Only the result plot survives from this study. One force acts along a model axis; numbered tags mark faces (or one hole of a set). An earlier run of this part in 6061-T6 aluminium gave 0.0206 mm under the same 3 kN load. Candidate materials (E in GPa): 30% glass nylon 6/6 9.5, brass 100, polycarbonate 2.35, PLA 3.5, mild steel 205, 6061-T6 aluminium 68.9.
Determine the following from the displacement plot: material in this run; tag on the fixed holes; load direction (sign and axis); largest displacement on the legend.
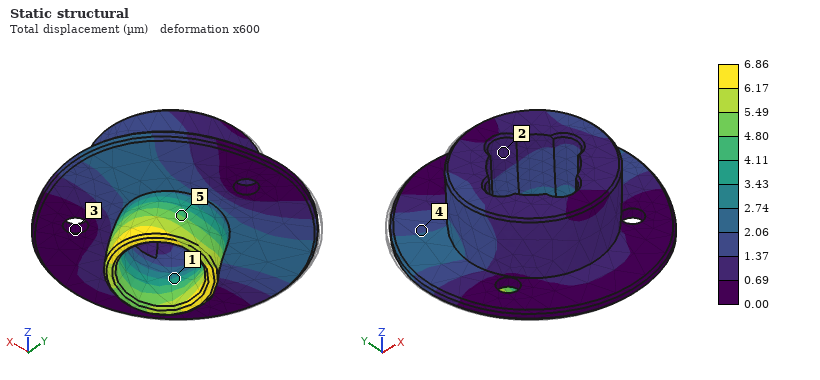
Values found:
mild steel
3
+X
6.86 µm
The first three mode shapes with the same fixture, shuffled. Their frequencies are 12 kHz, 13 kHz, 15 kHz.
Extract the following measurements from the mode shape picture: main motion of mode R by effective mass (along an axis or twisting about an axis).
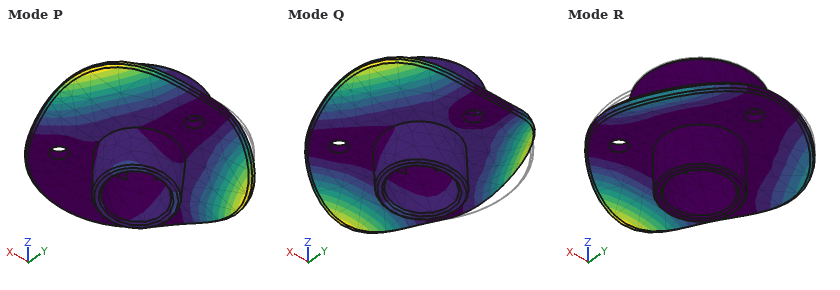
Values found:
along Z
